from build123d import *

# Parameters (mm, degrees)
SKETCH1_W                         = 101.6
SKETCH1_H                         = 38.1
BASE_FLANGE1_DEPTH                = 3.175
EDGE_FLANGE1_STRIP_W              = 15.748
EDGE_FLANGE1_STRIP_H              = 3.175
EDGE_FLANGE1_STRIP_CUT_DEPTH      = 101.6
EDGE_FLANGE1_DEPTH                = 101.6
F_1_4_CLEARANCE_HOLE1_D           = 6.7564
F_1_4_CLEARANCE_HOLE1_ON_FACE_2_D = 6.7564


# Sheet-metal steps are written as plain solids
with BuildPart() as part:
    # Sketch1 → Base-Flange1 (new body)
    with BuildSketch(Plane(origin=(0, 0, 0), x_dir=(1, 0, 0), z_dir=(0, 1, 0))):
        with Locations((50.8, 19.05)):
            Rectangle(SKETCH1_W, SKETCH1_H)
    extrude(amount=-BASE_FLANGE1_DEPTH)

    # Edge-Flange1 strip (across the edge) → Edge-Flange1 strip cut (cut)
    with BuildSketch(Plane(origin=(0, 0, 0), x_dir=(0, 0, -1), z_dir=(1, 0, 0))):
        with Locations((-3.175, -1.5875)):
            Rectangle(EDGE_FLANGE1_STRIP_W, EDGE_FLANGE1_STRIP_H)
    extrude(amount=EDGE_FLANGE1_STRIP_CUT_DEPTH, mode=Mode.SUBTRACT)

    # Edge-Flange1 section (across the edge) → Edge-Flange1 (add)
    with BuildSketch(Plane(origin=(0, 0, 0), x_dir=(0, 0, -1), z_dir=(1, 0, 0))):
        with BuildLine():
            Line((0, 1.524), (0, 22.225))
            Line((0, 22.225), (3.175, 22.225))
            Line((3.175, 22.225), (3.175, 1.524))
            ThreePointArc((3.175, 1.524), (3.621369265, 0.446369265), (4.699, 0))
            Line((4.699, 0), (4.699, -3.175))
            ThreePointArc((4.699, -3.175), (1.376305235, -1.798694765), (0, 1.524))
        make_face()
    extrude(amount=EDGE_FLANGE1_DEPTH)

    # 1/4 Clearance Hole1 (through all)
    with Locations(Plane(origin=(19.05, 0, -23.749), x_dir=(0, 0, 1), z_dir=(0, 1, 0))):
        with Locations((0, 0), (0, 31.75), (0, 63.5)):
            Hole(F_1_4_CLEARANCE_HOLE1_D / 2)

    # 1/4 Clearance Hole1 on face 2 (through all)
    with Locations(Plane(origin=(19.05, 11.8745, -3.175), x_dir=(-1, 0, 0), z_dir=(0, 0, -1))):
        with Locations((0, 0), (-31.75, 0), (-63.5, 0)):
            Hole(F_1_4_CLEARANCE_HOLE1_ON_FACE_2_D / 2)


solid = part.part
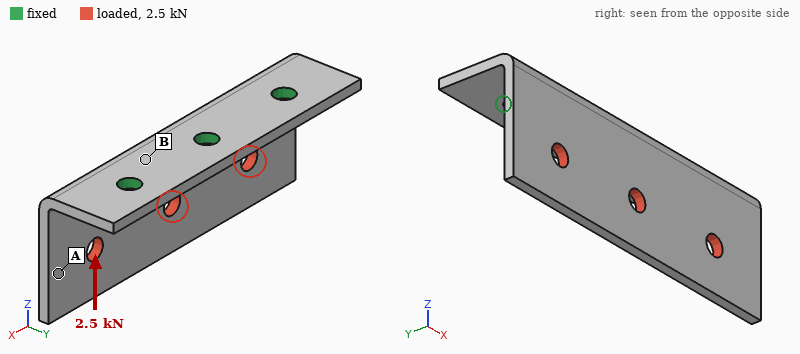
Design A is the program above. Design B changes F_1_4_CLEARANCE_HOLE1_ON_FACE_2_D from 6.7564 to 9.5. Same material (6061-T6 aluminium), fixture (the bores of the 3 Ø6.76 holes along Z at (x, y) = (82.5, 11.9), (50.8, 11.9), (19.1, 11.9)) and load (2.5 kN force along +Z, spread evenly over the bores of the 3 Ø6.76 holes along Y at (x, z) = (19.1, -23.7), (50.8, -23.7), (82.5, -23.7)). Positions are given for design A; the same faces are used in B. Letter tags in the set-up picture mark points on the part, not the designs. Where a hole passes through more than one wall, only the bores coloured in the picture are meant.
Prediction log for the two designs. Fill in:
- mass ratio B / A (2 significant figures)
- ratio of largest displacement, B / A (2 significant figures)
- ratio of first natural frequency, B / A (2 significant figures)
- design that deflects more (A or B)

0.98
0.74
1.1
A
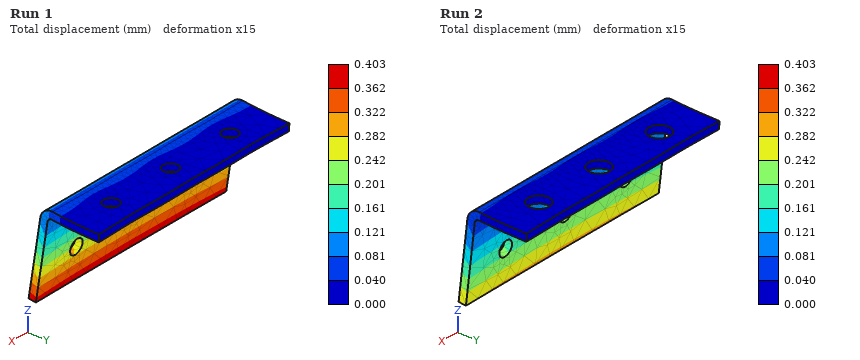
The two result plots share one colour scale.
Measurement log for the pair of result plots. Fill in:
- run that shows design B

Run 2
